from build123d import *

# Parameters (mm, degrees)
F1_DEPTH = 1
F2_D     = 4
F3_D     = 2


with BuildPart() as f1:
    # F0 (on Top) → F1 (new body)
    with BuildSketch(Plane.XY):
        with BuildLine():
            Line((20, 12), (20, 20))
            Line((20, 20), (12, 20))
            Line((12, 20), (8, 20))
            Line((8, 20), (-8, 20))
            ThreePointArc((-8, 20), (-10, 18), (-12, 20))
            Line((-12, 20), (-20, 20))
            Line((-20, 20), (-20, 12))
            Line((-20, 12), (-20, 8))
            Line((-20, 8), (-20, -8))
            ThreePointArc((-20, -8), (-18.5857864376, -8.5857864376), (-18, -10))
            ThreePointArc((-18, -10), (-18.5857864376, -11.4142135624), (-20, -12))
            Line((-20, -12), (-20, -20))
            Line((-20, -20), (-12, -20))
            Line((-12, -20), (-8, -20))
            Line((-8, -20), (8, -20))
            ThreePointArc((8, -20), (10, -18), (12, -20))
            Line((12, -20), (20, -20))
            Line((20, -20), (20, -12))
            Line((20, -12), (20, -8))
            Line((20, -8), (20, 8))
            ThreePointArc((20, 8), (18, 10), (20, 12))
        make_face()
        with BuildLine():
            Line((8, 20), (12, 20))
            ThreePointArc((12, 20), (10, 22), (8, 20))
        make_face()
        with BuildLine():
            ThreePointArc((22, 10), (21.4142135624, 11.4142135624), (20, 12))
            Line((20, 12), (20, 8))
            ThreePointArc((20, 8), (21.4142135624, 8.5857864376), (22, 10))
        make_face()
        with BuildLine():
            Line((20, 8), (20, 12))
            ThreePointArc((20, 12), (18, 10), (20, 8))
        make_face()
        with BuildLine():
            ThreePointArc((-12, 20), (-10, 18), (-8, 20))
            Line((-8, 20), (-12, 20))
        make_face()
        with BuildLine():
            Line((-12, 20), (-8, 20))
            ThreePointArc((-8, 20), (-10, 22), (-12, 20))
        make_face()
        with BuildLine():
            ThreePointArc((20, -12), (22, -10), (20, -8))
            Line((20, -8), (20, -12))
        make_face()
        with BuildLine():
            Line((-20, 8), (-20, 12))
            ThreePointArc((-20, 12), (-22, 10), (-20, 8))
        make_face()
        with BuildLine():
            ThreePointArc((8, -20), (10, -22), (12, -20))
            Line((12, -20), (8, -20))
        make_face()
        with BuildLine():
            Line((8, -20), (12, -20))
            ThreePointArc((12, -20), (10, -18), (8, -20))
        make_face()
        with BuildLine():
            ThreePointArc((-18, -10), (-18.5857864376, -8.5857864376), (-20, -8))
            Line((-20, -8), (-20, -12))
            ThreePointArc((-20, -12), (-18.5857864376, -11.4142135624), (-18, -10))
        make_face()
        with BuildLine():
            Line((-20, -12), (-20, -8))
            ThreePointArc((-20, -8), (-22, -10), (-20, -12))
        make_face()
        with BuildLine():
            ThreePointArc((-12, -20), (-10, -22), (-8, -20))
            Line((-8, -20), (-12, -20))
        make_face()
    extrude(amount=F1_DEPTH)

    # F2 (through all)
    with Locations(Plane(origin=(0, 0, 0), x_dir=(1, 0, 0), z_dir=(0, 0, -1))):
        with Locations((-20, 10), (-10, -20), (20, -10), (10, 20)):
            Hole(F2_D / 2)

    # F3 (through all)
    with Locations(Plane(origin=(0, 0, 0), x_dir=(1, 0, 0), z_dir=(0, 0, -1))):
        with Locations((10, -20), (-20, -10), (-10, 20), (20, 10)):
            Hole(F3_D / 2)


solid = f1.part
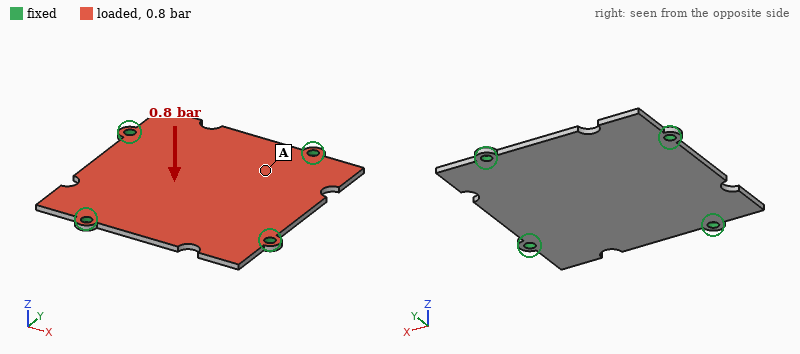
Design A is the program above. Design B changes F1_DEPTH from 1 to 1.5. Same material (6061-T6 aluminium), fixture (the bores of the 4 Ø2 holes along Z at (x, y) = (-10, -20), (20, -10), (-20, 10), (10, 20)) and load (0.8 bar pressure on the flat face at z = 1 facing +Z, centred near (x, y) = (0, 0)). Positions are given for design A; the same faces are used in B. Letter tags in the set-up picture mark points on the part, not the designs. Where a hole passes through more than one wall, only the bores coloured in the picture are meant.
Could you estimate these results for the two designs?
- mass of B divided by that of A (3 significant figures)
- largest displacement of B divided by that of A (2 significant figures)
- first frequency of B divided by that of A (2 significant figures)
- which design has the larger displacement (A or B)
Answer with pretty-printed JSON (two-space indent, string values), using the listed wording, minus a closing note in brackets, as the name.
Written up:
{
  "mass of B divided by that of A": "1.50",
  "largest displacement of B divided by that of A": "0.31",
  "first frequency of B divided by that of A": "1.5",
  "which design has the larger displacement": "A"
}
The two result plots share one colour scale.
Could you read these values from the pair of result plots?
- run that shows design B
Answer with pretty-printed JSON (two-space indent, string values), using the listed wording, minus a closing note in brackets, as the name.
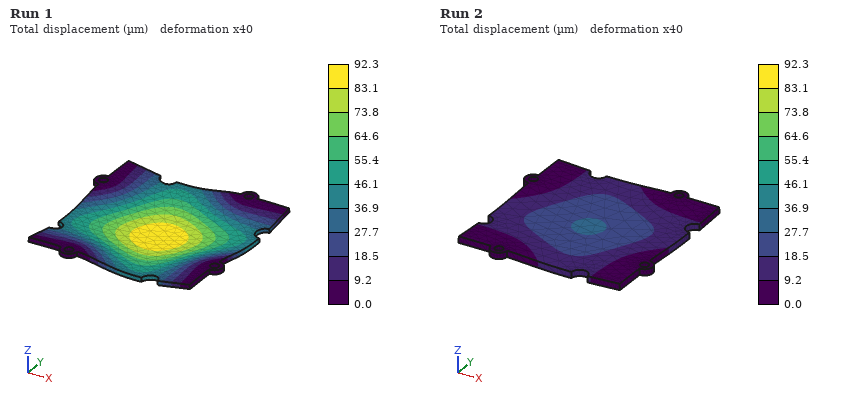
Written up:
{
  "run that shows design B": "Run 2"
}
